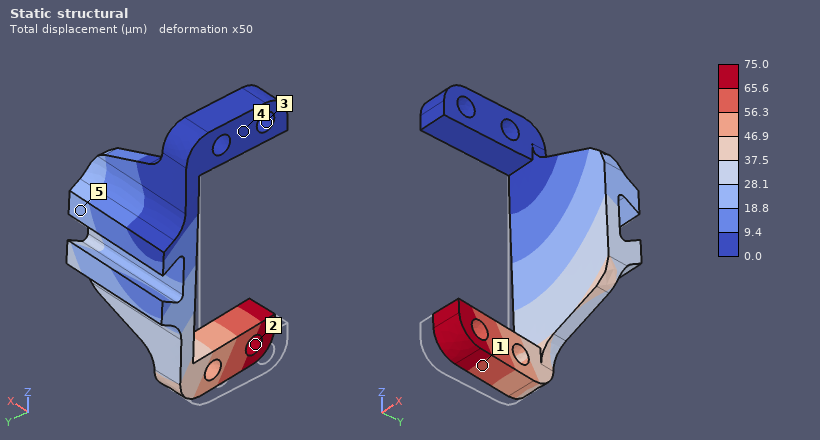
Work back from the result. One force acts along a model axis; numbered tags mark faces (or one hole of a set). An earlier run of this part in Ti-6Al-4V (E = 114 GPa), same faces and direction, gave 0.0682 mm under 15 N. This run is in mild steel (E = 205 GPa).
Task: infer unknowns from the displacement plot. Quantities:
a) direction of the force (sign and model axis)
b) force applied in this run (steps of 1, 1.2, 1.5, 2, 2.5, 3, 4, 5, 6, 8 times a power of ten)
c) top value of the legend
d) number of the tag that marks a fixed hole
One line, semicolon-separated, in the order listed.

+X; 30 N; 75.0 µm; 3
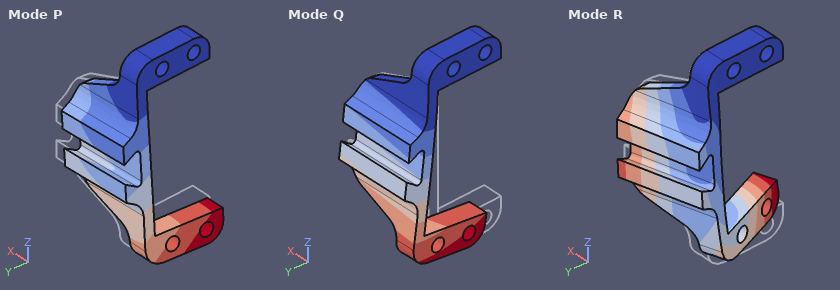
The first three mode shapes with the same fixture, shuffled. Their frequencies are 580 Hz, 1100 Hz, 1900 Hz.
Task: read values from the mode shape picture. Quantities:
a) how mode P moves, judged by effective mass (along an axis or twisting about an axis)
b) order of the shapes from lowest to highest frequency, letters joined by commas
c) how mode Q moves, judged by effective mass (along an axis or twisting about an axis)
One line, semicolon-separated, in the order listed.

along X; Q, P, R; along Y
